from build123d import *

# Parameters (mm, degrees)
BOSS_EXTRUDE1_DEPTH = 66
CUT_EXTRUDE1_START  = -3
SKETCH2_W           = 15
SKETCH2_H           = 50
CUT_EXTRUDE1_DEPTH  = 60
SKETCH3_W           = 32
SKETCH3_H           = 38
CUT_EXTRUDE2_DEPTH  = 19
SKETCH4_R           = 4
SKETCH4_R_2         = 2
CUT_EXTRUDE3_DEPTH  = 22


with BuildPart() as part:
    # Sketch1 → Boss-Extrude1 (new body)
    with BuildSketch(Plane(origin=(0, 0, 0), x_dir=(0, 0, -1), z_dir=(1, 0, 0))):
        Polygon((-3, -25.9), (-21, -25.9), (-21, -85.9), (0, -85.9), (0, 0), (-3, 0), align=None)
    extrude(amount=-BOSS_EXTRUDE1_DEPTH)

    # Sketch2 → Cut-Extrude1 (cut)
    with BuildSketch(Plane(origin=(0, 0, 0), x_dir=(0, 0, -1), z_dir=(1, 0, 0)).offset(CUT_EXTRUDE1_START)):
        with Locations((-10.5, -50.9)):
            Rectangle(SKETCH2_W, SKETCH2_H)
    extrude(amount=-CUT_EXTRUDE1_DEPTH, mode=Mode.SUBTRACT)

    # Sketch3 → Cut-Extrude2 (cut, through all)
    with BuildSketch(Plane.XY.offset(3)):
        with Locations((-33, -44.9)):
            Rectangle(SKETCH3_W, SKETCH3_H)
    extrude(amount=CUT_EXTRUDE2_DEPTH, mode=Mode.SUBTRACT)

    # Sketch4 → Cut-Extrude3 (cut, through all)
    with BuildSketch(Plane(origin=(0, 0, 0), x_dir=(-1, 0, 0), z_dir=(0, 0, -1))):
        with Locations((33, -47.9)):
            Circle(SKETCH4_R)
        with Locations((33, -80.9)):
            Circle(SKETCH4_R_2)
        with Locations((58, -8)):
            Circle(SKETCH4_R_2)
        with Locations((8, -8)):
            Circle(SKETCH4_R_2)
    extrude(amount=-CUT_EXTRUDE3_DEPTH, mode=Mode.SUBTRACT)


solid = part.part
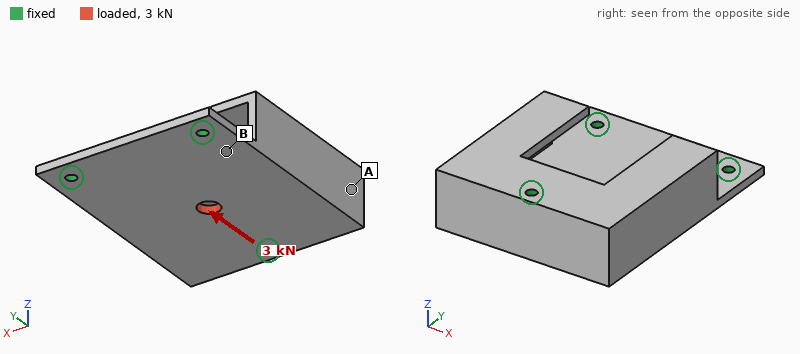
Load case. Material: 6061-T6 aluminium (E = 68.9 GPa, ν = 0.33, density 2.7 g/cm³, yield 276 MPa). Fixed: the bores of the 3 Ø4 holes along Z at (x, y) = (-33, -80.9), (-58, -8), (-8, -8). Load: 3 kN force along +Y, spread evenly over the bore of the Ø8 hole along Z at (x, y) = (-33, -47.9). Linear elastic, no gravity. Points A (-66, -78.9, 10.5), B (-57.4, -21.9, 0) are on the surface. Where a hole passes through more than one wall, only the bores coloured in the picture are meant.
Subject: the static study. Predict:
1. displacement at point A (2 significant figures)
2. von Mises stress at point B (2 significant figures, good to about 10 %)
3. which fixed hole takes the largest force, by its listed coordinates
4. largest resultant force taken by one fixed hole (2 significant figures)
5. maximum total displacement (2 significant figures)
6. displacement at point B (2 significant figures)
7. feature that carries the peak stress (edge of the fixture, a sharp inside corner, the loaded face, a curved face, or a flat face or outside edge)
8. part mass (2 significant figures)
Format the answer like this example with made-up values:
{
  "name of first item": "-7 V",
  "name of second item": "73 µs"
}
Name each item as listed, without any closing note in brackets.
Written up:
{
  "displacement at point A": "3.6 µm",
  "von Mises stress at point B": "13 MPa",
  "which fixed hole takes the largest force, by its listed coordinates": "(-33, -80.9)",
  "largest resultant force taken by one fixed hole": "1.5 kN",
  "maximum total displacement": "13 µm",
  "displacement at point B": "3.3 µm",
  "feature that carries the peak stress": "the loaded face",
  "part mass": "110 g"
}
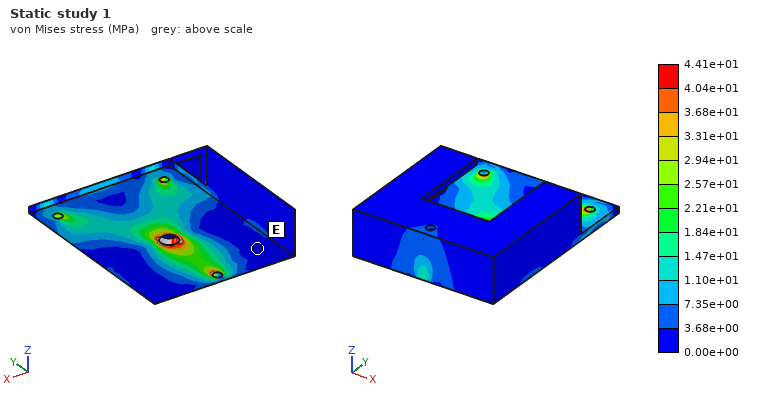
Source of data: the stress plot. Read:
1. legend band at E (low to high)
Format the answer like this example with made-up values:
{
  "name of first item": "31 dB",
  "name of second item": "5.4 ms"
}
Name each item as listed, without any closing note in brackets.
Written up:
{
  "legend band at E": "0.00e+00 to 3.68e+00 MPa"
}
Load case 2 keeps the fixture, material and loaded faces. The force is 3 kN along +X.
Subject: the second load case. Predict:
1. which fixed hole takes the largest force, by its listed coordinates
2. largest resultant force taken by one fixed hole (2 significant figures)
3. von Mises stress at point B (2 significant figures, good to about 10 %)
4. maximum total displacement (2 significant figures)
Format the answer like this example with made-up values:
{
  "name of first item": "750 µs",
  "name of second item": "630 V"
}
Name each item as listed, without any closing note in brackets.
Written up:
{
  "which fixed hole takes the largest force, by its listed coordinates": "(-33, -80.9)",
  "largest resultant force taken by one fixed hole": "1.4 kN",
  "von Mises stress at point B": "14 MPa",
  "maximum total displacement": "18 µm"
}
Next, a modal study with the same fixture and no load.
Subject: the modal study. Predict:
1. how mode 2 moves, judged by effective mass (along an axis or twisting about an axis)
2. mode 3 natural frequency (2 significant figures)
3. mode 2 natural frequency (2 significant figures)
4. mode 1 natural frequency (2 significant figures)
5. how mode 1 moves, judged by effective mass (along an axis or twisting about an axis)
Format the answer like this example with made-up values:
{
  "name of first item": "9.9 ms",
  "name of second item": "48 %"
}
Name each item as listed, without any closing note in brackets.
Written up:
{
  "how mode 2 moves, judged by effective mass": "twisting about Y",
  "mode 3 natural frequency": "5200 Hz",
  "mode 2 natural frequency": "3800 Hz",
  "mode 1 natural frequency": "3400 Hz",
  "how mode 1 moves, judged by effective mass": "along Z"
}
